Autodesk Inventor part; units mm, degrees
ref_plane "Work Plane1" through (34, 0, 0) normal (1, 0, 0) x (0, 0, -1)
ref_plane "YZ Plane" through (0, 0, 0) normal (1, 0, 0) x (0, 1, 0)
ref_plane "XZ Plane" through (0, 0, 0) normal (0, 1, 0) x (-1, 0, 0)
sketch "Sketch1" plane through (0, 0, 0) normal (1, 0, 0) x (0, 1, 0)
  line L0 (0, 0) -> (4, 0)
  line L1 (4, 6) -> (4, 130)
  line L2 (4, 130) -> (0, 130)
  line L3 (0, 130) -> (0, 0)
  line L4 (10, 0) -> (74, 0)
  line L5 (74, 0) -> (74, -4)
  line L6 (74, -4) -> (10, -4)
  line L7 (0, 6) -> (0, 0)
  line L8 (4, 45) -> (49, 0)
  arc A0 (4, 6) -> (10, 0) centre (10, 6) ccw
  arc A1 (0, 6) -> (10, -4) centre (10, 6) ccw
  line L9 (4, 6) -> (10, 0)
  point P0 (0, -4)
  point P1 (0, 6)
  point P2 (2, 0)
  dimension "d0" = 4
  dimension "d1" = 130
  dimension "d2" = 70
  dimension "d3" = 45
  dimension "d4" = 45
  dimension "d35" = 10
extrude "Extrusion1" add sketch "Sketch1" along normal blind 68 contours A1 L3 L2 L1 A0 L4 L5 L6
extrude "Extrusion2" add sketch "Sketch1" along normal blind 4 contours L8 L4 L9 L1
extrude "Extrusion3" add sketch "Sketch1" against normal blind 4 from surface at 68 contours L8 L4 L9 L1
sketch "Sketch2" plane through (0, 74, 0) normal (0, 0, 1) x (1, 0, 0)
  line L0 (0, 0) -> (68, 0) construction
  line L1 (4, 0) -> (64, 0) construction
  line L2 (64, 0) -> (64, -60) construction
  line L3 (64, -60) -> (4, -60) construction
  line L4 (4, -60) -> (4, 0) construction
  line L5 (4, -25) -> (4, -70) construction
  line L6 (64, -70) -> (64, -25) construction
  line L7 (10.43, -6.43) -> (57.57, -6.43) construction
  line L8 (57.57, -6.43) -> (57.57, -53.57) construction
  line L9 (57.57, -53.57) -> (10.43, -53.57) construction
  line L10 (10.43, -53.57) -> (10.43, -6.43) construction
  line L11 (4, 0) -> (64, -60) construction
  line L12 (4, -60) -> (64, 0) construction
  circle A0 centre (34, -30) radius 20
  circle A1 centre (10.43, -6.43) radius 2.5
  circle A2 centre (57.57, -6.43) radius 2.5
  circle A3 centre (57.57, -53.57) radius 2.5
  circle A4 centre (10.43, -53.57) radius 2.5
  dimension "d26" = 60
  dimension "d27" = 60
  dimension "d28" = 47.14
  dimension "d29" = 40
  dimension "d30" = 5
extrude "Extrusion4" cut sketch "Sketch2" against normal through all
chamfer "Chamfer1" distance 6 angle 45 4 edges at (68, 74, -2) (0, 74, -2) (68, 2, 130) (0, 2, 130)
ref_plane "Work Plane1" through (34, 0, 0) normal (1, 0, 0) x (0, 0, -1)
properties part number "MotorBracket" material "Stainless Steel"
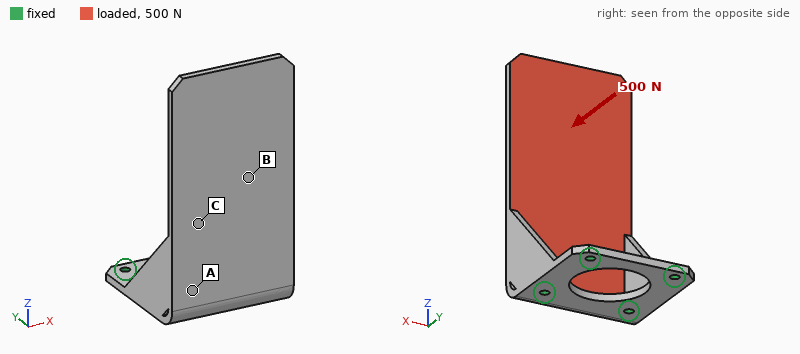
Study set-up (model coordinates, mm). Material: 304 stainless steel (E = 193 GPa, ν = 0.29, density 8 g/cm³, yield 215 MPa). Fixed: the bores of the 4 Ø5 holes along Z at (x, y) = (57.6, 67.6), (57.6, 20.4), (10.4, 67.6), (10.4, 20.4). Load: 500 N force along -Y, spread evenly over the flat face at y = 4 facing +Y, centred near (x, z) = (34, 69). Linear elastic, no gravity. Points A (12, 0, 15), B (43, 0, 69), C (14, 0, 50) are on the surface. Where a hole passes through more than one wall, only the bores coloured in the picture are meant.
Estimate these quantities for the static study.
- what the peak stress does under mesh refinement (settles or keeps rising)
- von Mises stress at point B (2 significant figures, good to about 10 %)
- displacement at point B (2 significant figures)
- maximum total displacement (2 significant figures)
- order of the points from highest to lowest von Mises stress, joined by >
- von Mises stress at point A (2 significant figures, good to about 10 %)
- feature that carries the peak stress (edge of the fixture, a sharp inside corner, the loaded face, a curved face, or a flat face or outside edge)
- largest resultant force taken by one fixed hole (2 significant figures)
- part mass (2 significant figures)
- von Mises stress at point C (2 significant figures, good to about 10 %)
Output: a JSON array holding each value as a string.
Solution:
["keeps rising", "51 MPa", "0.23 mm", "0.81 mm", "C > B > A", "17 MPa", "edge of the fixture", "390 N", "460 g", "79 MPa"]
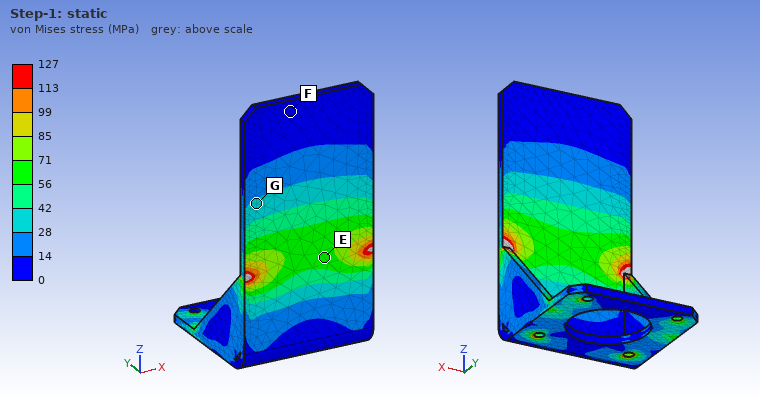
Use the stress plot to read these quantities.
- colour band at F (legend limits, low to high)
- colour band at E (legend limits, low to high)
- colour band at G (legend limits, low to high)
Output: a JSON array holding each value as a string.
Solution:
["0 to 14 MPa", "56 to 71 MPa", "28 to 42 MPa"]
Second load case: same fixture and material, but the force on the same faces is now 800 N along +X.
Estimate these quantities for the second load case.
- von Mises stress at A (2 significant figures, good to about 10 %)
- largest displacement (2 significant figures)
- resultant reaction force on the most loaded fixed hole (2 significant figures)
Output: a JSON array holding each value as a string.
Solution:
["13 MPa", "0.12 mm", "1.4 kN"]
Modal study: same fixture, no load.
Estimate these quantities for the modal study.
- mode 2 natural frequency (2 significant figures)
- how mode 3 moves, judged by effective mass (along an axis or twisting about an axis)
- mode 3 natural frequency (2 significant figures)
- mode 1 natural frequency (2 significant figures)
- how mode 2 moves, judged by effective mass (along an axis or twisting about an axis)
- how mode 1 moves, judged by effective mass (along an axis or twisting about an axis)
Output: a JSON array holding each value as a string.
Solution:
["890 Hz", "along X", "1300 Hz", "310 Hz", "along X", "along Y"]
